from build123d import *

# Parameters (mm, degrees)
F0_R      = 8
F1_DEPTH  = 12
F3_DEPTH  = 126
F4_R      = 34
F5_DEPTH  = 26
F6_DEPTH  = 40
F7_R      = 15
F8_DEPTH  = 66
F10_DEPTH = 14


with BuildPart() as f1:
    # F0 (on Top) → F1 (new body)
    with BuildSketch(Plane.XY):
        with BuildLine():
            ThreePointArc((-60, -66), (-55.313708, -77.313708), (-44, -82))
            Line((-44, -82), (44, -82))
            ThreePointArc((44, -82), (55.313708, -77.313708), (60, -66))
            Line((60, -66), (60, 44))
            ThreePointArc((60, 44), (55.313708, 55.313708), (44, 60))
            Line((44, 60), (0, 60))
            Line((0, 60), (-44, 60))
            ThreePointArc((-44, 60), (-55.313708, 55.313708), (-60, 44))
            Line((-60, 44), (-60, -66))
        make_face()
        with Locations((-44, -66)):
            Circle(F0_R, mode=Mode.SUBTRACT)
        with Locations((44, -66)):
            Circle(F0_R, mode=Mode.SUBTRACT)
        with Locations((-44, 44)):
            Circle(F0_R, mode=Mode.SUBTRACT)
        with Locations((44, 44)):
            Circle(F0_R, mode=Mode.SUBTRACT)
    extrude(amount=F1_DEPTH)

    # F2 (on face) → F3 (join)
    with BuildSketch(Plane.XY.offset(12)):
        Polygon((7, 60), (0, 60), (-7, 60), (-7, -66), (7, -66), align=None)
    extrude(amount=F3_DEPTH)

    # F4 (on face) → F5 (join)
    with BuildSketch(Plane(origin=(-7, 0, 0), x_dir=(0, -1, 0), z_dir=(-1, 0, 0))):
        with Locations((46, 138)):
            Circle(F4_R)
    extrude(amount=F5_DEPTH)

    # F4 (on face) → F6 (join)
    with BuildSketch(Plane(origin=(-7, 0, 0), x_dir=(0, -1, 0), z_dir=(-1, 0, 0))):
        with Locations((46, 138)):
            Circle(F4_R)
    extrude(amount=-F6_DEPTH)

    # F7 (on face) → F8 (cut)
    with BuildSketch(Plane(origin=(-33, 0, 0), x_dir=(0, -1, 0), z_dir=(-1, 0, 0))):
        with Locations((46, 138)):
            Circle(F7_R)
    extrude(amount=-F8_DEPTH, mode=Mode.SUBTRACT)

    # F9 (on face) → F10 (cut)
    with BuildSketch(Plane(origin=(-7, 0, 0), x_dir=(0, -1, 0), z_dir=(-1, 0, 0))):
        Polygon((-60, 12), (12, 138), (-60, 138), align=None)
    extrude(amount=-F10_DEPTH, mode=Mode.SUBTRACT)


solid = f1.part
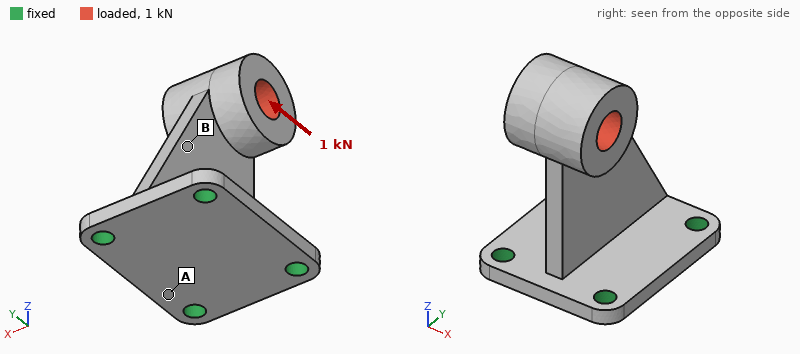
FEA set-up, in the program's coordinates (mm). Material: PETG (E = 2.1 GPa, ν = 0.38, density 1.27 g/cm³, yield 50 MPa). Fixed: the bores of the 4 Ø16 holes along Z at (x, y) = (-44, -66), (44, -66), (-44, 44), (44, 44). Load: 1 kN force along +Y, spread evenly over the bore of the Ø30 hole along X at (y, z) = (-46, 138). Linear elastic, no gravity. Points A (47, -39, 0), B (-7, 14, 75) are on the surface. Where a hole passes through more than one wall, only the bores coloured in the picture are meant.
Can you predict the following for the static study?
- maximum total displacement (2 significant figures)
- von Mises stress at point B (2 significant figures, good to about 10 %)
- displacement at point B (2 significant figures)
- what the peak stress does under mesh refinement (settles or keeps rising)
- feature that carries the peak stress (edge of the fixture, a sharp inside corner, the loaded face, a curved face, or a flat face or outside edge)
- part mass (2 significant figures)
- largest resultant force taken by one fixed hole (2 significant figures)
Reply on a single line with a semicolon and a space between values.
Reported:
1.4 mm; 3.3 MPa; 0.47 mm; keeps rising; edge of the fixture; 660 g; 700 N
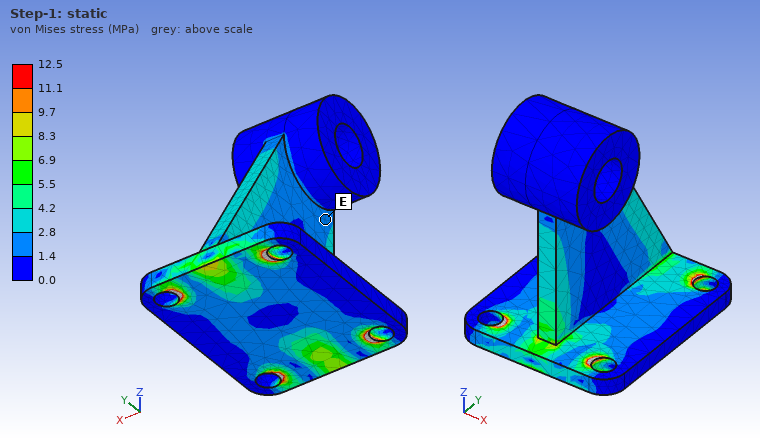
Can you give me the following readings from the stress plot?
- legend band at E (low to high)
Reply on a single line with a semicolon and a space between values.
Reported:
1.4 to 2.8 MPa
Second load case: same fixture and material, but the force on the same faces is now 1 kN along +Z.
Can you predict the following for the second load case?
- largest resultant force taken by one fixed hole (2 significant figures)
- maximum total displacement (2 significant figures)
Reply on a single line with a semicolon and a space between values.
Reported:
420 N; 0.45 mm
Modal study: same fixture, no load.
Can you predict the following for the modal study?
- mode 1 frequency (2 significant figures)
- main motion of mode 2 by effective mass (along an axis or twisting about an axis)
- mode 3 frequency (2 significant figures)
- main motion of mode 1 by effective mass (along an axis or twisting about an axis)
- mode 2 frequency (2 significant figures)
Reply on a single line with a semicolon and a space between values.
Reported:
72 Hz; along Y; 300 Hz; along X; 280 Hz
